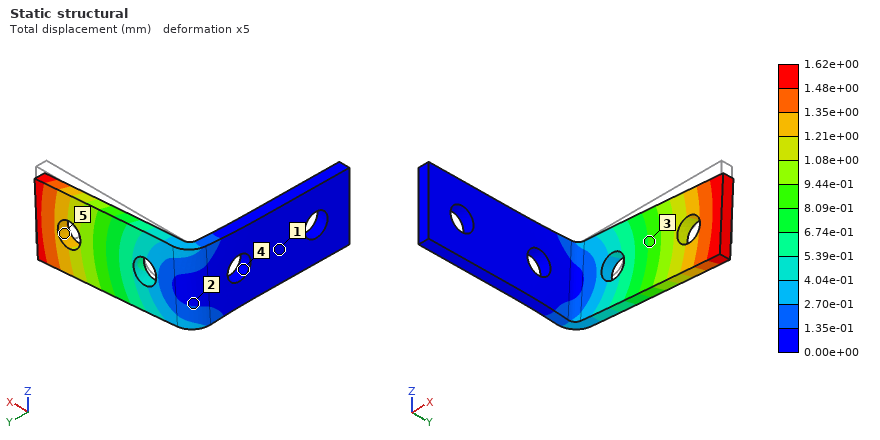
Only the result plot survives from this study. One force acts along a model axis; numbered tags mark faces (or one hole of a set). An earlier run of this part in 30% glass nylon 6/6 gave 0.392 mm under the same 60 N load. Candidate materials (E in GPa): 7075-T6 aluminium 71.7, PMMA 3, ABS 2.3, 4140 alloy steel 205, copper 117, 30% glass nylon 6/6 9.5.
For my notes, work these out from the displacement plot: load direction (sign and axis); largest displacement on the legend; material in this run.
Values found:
-Z
1.62e+00 mm
ABS
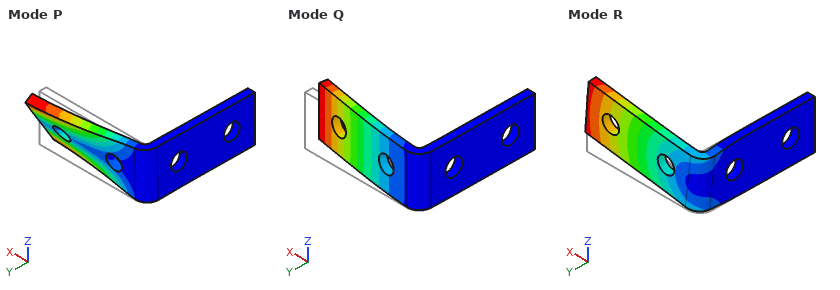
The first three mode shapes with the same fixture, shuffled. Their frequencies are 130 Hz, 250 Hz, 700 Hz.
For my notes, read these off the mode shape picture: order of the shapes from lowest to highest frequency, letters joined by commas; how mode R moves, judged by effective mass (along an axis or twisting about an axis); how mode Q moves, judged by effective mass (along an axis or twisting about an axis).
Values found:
Q, R, P
along Z
along Y
